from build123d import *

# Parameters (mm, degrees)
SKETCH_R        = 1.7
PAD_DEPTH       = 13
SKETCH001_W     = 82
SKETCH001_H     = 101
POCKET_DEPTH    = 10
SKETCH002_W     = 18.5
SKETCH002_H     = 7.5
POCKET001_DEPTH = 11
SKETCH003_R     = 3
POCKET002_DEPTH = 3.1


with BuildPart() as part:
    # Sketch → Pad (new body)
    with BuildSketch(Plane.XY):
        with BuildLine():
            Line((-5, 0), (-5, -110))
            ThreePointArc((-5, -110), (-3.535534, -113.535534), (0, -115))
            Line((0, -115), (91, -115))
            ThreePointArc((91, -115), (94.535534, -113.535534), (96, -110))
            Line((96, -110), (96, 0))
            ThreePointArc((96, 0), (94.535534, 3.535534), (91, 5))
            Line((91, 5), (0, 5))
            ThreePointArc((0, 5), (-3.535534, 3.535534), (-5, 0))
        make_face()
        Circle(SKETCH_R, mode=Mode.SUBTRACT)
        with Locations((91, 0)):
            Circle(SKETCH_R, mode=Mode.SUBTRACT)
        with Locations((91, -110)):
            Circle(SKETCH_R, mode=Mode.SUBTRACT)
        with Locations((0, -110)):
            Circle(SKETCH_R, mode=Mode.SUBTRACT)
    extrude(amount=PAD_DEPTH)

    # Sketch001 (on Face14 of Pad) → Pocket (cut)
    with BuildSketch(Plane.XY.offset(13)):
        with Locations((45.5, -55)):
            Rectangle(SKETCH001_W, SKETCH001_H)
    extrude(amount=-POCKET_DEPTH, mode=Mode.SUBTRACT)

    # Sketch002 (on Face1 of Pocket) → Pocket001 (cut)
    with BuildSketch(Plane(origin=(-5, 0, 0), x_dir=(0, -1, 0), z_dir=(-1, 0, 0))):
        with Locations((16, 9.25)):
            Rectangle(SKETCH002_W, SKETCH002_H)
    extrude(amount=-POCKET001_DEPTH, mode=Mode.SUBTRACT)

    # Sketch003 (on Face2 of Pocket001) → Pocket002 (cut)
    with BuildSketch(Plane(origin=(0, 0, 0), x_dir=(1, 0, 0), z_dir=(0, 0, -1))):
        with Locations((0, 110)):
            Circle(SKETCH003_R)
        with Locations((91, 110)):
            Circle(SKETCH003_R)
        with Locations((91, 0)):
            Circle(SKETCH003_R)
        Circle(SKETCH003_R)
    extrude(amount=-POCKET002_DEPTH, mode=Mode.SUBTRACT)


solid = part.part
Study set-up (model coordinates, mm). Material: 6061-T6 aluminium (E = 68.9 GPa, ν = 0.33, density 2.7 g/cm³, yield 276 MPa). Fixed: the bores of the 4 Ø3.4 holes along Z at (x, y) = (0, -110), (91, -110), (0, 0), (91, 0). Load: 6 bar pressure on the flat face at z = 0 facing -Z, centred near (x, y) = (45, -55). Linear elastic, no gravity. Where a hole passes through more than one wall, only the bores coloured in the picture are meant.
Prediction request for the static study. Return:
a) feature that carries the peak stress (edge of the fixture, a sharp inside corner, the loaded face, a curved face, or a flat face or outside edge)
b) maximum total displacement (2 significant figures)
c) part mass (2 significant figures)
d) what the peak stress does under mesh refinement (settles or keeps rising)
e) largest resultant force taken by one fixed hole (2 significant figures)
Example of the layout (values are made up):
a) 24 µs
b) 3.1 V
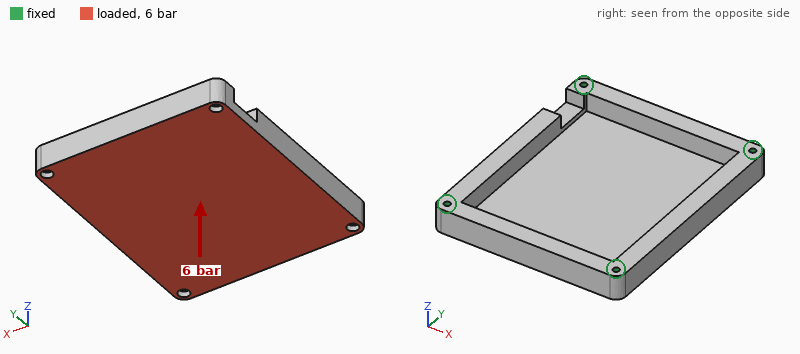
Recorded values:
a) edge of the fixture
b) 0.53 mm
c) 200 g
d) keeps rising
e) 2.9 kN
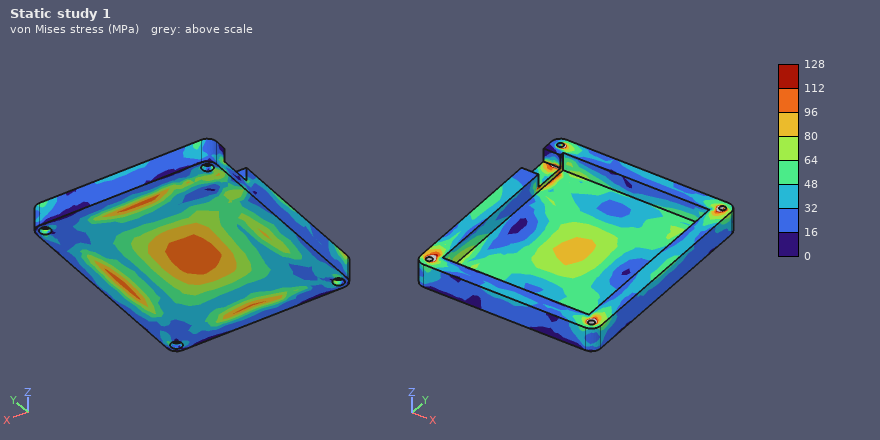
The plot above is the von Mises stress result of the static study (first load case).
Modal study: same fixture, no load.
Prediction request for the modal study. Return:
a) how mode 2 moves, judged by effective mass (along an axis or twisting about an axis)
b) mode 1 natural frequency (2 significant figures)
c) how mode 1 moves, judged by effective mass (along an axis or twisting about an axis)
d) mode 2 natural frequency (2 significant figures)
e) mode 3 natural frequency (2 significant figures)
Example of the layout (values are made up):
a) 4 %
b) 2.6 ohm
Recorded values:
a) twisting about Y
b) 2400 Hz
c) along Z
d) 3700 Hz
e) 4500 Hz
